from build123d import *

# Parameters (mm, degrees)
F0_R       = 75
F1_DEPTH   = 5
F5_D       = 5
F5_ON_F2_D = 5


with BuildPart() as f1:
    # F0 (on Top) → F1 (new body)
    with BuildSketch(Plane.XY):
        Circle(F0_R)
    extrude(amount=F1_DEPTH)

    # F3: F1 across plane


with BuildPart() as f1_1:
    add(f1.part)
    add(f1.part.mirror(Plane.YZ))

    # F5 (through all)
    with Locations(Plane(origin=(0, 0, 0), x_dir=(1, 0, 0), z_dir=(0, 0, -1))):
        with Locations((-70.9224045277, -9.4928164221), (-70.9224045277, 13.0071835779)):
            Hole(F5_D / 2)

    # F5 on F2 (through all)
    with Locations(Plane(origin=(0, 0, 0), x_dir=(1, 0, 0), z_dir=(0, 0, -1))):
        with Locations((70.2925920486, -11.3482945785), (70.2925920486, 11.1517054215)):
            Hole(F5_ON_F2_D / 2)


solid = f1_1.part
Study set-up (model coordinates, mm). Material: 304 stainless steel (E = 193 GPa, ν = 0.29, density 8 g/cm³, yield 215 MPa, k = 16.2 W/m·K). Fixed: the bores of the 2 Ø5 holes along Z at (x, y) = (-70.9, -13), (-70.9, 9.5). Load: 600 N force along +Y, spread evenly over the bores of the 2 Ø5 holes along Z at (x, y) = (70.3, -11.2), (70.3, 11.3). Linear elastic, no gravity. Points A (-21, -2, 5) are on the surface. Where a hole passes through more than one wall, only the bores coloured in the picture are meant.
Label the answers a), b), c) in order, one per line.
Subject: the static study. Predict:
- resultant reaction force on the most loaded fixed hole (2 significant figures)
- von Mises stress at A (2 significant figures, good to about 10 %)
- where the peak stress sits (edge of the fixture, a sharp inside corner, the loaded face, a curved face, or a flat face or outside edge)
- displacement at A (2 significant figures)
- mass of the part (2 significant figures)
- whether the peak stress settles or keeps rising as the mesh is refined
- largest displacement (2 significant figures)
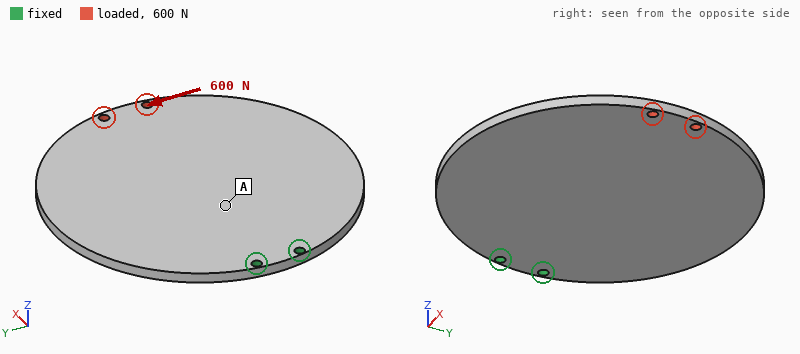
a) 3.2 kN
b) 6.3 MPa
c) edge of the fixture
d) 19 µm
e) 700 g
f) keeps rising
g) 59 µm
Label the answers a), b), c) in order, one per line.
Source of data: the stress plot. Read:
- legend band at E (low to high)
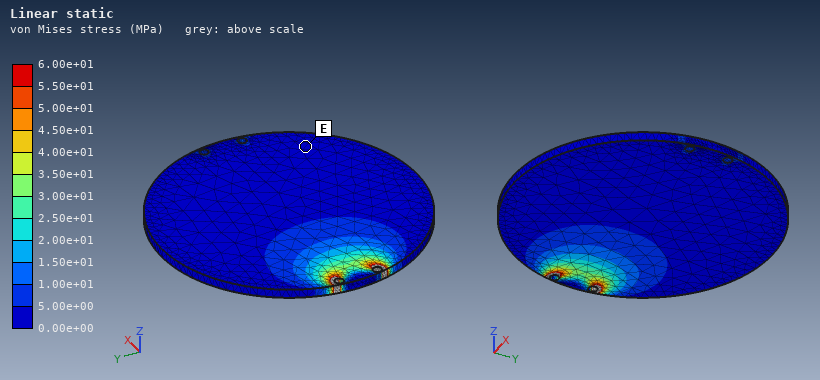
a) 0.00e+00 to 5.00e+00 MPa
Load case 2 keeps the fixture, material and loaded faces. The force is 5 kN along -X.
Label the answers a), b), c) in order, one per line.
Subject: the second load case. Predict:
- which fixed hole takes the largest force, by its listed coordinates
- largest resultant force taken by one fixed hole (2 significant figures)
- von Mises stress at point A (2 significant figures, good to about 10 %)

a) (-70.9, 9.5)
b) 2.9 kN
c) 15 MPa
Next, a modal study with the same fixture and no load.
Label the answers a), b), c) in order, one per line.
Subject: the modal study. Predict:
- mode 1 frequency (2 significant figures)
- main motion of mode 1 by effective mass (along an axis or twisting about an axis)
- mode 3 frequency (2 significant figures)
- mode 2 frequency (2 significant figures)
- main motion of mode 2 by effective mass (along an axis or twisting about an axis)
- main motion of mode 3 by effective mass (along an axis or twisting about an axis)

a) 160 Hz
b) along Z
c) 910 Hz
d) 360 Hz
e) twisting about X
f) along Z
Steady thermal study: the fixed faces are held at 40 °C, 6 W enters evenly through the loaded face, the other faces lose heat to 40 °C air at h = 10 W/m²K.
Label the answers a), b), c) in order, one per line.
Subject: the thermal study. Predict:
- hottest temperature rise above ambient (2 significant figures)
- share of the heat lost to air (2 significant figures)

a) 64 K
b) 87 %
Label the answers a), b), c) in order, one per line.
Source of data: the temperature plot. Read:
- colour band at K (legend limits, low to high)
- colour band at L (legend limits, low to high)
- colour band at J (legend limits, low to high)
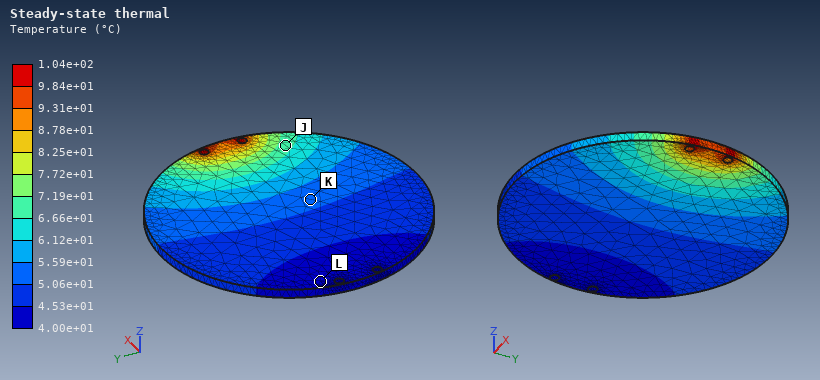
a) 5.06e+01 to 5.59e+01 °C
b) 4.00e+01 to 4.53e+01 °C
c) 6.66e+01 to 7.19e+01 °C
